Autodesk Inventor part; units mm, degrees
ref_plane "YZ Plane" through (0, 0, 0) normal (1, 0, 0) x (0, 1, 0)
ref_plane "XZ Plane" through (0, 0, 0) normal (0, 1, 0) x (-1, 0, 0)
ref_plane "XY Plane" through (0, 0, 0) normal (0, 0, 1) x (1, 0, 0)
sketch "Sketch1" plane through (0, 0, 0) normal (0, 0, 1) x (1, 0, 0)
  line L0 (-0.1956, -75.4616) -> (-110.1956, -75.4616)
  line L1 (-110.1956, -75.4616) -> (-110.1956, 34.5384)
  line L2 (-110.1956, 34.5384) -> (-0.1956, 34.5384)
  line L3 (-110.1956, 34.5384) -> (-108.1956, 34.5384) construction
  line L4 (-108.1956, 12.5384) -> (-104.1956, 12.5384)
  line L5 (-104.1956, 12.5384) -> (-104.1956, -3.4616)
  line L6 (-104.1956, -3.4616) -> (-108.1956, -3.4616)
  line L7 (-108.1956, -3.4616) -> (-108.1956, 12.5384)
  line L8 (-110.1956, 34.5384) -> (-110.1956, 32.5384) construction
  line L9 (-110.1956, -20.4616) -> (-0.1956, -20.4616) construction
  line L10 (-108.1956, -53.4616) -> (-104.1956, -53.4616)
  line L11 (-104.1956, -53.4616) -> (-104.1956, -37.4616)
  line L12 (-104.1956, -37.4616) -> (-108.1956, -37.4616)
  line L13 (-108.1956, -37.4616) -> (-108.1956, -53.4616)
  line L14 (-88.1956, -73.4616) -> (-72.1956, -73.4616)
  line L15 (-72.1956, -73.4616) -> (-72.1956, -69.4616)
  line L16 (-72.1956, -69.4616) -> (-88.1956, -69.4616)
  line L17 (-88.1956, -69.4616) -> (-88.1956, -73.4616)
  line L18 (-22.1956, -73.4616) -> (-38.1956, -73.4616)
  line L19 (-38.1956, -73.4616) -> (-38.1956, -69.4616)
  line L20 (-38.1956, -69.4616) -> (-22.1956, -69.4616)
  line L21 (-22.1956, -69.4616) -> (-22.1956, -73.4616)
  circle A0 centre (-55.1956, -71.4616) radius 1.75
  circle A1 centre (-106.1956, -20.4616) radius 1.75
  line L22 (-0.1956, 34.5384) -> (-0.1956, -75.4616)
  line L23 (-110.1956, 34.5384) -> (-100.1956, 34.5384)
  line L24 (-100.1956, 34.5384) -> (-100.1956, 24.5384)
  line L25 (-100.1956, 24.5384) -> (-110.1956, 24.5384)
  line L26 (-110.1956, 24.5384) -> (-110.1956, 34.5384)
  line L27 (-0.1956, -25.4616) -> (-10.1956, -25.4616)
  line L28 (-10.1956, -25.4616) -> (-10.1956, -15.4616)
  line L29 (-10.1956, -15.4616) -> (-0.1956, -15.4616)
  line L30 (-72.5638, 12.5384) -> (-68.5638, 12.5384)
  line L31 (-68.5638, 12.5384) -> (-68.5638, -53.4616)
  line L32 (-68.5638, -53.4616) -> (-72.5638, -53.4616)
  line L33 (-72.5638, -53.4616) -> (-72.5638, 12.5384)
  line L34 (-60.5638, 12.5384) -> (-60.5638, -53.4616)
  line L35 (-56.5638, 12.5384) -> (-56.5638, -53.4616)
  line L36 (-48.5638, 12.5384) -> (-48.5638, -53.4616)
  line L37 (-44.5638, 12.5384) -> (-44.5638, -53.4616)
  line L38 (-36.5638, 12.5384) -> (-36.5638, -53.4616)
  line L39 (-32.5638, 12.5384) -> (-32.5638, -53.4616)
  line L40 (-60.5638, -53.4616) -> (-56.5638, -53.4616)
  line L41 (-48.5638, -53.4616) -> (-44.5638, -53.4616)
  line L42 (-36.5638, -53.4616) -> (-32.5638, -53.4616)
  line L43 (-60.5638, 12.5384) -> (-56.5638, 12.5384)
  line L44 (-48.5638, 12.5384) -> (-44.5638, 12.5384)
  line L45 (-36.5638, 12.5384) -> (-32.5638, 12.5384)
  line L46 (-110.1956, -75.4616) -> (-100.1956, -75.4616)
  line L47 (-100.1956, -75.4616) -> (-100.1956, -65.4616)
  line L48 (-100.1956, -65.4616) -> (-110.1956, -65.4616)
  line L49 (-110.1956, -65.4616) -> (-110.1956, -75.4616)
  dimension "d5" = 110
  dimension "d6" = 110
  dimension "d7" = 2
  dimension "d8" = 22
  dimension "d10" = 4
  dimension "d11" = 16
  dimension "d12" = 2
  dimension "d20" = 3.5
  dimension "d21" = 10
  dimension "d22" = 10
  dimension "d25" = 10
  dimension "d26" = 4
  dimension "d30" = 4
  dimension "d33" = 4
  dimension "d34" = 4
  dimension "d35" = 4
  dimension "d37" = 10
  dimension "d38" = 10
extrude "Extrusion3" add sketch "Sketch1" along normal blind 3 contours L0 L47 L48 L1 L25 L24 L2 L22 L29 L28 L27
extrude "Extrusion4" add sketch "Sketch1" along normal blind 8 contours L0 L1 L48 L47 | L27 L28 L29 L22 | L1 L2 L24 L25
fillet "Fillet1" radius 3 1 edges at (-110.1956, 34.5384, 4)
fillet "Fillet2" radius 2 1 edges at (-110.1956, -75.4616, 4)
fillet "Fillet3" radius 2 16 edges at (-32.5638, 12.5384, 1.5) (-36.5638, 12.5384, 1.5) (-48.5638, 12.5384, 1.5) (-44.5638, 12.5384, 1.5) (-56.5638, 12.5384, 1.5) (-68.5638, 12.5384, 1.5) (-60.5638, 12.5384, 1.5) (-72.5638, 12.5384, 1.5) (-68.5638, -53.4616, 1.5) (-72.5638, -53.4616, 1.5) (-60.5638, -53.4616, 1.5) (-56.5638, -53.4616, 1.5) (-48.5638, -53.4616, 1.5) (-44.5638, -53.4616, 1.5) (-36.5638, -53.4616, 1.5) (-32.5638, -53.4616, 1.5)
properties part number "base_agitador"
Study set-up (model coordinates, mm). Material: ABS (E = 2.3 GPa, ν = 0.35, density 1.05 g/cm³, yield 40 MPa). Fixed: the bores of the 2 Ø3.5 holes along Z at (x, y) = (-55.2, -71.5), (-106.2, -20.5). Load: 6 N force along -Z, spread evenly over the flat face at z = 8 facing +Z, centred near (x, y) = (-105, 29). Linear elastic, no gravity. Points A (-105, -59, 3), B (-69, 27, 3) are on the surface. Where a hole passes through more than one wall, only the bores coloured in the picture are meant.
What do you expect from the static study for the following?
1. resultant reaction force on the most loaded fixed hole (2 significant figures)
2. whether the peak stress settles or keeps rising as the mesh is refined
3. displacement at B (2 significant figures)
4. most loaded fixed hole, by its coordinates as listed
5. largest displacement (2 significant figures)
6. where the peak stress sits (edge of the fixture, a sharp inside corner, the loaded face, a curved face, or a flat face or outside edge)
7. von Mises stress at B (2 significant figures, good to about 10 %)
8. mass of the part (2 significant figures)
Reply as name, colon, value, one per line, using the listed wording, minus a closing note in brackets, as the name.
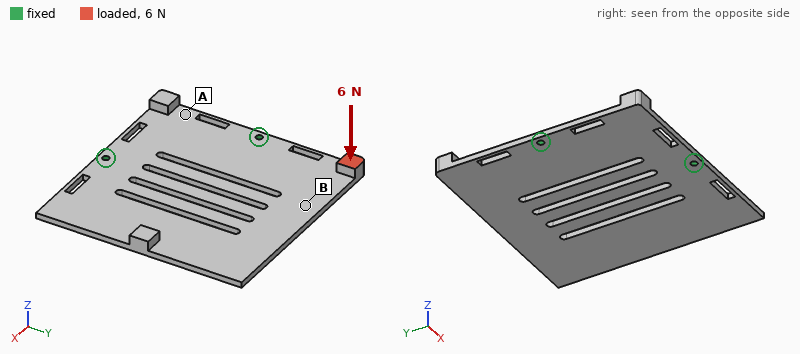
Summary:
resultant reaction force on the most loaded fixed hole: 7.9 N
whether the peak stress settles or keeps rising as the mesh is refined: keeps rising
displacement at B: 1.1 mm
most loaded fixed hole, by its coordinates as listed: (-106.2, -20.5)
largest displacement: 1.6 mm
where the peak stress sits: edge of the fixture
von Mises stress at B: 1.5 MPa
mass of the part: 36 g
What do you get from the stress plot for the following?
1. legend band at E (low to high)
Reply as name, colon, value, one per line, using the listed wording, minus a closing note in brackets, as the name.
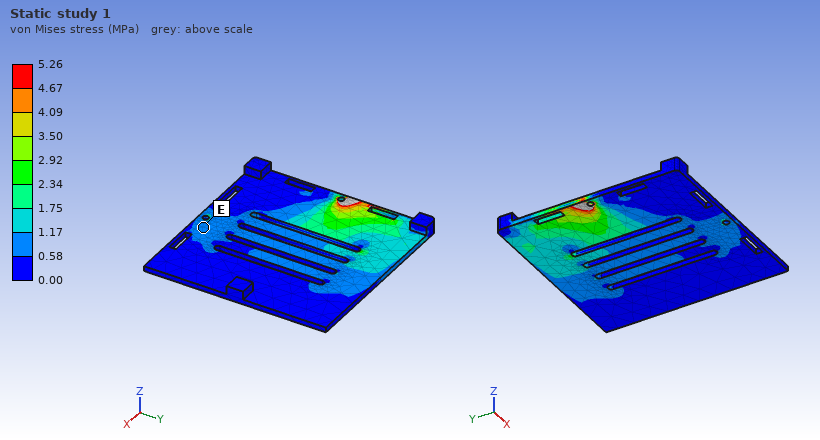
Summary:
legend band at E: 0.58 to 1.17 MPa
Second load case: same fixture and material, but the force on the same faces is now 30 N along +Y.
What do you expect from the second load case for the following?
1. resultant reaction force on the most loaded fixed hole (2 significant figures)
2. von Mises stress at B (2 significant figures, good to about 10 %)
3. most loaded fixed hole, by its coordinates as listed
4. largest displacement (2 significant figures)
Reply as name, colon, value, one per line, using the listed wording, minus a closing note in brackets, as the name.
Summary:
resultant reaction force on the most loaded fixed hole: 30 N
von Mises stress at B: 1.8 MPa
most loaded fixed hole, by its coordinates as listed: (-106.2, -20.5)
largest displacement: 1.5 mm
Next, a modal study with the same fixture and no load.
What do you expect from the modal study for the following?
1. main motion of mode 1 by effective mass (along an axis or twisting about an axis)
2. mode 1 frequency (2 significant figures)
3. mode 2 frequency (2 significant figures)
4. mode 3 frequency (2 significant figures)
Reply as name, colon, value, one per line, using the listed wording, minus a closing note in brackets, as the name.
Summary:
main motion of mode 1 by effective mass: along Z
mode 1 frequency: 64 Hz
mode 2 frequency: 160 Hz
mode 3 frequency: 280 Hz
